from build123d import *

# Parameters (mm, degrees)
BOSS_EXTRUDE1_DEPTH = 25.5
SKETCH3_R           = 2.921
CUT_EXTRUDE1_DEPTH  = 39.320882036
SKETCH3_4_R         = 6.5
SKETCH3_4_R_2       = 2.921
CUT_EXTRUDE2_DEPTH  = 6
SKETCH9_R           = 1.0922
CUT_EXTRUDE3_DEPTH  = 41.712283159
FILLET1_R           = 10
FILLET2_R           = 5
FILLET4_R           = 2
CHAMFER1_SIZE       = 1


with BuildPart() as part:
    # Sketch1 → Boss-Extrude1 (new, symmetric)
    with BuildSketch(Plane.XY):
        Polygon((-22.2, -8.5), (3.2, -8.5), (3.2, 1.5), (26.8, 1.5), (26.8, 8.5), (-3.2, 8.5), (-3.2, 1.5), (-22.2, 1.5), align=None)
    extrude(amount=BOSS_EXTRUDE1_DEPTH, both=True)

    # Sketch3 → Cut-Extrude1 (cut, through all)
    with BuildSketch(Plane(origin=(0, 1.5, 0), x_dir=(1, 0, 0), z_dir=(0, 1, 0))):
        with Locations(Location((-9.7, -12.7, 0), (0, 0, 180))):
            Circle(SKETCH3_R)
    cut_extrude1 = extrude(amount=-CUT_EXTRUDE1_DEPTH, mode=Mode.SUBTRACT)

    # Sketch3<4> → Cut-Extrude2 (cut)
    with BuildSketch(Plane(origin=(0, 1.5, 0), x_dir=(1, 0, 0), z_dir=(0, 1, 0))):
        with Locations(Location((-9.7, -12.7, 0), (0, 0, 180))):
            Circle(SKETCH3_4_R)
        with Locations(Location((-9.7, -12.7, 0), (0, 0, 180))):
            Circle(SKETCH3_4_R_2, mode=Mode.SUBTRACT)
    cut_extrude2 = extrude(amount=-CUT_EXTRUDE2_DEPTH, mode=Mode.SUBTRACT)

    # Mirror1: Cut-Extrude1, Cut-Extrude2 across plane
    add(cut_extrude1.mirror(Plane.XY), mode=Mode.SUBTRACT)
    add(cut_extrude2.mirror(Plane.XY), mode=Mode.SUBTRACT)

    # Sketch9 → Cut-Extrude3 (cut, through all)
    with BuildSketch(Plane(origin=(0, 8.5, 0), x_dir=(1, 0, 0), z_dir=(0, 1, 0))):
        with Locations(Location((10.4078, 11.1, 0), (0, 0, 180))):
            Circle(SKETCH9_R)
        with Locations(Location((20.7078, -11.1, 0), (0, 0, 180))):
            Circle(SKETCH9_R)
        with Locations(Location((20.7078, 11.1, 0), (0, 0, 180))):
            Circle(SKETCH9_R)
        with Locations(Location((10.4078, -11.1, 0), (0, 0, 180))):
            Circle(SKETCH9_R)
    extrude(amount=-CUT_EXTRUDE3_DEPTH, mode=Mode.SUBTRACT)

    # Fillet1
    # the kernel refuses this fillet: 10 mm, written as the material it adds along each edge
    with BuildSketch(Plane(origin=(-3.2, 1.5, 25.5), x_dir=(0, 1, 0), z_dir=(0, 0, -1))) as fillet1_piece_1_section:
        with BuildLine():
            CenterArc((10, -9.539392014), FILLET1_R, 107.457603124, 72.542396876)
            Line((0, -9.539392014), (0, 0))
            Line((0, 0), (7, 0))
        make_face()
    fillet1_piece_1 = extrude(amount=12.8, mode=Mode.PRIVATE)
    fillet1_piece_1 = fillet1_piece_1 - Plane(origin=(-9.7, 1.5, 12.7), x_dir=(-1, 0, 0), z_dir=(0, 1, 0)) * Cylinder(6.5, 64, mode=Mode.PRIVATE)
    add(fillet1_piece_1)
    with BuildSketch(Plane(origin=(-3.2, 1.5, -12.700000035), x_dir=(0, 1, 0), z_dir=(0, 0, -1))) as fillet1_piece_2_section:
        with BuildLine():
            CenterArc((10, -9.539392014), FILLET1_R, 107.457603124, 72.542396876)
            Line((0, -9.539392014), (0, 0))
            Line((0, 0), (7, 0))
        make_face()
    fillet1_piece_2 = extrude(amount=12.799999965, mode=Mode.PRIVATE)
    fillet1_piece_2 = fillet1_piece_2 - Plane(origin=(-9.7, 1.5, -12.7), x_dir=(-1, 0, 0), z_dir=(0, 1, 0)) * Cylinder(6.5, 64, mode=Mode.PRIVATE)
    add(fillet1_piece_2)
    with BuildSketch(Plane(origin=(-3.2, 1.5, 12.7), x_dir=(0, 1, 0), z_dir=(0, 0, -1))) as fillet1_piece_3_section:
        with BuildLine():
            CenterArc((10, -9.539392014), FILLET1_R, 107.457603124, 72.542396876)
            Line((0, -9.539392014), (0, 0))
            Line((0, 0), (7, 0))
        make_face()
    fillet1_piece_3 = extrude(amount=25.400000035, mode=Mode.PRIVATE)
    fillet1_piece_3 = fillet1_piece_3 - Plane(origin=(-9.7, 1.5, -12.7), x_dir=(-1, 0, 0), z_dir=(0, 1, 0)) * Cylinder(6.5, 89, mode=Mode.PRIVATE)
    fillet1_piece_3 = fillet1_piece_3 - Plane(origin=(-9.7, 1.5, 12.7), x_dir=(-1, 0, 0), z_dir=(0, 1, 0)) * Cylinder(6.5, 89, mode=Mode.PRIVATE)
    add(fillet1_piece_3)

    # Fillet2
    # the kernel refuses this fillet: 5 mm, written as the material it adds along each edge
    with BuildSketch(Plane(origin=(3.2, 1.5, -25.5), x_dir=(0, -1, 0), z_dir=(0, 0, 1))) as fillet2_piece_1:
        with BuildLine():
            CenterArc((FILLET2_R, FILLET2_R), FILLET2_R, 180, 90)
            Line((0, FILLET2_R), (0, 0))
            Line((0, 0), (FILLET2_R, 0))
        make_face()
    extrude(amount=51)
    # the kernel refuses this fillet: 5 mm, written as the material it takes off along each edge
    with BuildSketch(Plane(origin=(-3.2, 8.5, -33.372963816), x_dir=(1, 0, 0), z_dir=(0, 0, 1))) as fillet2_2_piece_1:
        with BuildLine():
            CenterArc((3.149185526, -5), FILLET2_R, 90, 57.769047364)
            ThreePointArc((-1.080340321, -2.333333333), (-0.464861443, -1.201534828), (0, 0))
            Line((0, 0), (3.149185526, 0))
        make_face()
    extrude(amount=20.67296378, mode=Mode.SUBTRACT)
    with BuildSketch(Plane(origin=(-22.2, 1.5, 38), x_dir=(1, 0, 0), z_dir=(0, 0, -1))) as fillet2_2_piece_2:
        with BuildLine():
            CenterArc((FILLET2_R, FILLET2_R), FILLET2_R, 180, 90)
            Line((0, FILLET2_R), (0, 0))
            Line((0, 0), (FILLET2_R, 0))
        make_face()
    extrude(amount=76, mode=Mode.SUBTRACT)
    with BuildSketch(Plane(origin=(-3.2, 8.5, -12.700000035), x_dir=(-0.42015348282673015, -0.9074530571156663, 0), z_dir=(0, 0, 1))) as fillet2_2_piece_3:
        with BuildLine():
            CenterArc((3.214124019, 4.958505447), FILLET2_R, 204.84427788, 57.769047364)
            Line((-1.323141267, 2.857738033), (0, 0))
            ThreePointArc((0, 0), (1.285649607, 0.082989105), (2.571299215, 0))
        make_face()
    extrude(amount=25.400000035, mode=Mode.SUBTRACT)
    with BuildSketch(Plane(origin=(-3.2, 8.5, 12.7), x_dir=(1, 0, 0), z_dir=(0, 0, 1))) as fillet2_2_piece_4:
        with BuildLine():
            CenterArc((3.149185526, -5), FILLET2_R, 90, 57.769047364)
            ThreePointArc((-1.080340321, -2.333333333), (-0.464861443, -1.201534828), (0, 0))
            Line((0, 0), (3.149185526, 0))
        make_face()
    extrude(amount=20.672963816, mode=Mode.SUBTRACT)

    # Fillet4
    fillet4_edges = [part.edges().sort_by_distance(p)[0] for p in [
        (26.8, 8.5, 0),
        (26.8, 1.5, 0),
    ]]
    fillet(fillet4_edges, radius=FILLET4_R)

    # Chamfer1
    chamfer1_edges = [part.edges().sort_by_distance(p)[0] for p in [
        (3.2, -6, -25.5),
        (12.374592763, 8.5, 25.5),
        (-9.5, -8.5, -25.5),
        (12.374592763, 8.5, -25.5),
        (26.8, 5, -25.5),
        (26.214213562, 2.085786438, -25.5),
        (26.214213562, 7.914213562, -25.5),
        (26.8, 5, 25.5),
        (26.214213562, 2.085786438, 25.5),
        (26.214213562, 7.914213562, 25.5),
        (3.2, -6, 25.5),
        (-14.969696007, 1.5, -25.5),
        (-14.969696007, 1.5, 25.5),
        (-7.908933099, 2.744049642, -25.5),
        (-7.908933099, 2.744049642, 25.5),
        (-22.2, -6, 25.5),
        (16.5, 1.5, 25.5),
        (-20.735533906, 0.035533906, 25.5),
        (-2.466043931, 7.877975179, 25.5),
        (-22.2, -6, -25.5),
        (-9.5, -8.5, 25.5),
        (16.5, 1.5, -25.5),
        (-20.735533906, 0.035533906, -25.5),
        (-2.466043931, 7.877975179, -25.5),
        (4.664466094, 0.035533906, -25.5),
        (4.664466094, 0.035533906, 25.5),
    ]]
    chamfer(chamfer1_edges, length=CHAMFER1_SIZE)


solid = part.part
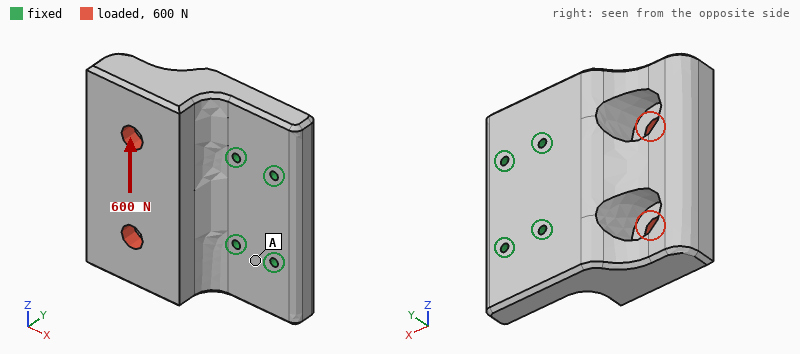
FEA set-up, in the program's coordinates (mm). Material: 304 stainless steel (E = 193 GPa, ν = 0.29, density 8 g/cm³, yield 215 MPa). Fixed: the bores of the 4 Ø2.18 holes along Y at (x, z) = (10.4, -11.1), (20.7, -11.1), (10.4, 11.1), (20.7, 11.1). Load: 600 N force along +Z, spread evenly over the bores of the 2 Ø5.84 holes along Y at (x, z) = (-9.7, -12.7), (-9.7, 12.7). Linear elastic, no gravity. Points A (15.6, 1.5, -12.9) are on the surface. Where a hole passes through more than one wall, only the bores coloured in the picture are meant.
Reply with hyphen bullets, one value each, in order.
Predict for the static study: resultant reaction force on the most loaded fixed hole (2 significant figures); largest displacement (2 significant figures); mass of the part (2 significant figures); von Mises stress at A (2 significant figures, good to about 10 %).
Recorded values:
- 540 N
- 2.3 µm
- 180 g
- 2.4 MPa
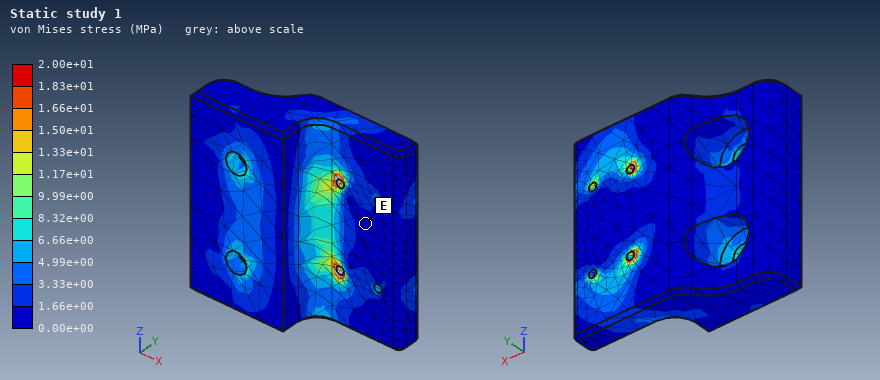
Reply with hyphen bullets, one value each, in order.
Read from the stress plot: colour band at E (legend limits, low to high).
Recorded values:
- 0.00e+00 to 1.66e+00 MPa
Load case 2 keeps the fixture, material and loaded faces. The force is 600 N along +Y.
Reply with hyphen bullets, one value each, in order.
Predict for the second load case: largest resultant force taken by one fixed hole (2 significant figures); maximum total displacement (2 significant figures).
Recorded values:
- 540 N
- 14 µm
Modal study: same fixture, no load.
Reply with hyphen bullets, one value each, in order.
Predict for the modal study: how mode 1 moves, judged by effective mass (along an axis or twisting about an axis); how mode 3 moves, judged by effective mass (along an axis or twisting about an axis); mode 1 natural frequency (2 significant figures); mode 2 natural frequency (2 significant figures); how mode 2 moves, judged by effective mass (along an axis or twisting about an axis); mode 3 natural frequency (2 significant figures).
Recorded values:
- along Y
- along Z
- 4000 Hz
- 7700 Hz
- twisting about X
- 10 kHz
